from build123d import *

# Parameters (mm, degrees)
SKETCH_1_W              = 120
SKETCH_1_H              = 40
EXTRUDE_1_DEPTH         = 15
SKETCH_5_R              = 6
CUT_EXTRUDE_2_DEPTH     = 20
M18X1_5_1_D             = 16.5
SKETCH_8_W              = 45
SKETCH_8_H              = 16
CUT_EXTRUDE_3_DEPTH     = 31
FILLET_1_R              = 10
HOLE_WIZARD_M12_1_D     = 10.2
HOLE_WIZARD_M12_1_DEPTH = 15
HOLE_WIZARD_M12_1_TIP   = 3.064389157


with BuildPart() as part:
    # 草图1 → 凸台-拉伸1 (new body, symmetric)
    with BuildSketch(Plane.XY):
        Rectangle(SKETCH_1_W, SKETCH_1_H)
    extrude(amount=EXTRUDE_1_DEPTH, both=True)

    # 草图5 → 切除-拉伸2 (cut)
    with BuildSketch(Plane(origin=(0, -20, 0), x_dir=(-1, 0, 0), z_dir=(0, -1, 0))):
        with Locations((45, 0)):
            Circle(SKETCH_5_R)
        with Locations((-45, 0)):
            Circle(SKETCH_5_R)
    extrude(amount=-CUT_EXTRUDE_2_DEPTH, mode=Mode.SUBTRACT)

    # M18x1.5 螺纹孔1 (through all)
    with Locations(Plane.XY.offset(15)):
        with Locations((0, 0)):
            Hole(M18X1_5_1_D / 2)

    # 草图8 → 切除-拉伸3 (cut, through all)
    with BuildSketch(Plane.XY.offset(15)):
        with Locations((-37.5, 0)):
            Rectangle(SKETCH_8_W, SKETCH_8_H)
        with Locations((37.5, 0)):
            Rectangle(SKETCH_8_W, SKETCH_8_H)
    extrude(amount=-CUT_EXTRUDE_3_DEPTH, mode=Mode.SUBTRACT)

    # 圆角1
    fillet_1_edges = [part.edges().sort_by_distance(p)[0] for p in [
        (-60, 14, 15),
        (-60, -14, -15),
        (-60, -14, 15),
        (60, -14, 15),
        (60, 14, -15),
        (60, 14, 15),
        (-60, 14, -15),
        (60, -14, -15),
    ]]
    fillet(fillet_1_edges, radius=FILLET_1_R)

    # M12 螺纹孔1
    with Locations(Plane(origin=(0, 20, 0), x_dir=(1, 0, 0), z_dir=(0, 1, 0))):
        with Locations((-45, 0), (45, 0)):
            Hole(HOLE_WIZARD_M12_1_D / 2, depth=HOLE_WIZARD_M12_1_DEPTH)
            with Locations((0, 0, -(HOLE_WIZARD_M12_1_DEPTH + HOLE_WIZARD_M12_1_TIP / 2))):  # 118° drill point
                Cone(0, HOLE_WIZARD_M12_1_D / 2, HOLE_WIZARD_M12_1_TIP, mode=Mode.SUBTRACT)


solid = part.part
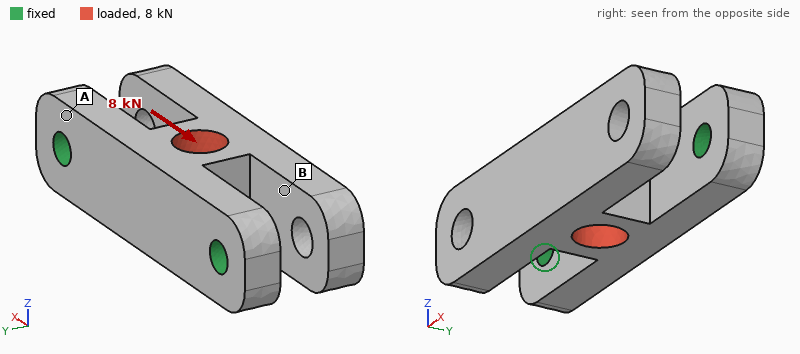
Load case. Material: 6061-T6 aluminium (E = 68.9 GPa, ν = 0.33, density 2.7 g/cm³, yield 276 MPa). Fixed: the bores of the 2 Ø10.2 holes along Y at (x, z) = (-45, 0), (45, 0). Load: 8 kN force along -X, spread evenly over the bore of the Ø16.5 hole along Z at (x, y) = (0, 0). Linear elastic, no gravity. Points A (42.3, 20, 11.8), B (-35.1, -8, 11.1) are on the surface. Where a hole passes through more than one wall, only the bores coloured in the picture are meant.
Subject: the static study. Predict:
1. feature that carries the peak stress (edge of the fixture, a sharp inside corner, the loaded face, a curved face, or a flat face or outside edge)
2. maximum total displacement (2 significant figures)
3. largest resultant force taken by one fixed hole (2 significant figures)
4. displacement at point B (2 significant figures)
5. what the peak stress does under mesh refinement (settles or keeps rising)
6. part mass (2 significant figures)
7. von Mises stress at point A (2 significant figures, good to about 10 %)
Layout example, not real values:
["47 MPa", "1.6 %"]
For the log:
["edge of the fixture", "73 µm", "4.4 kN", "48 µm", "keeps rising", "240 g", "16 MPa"]
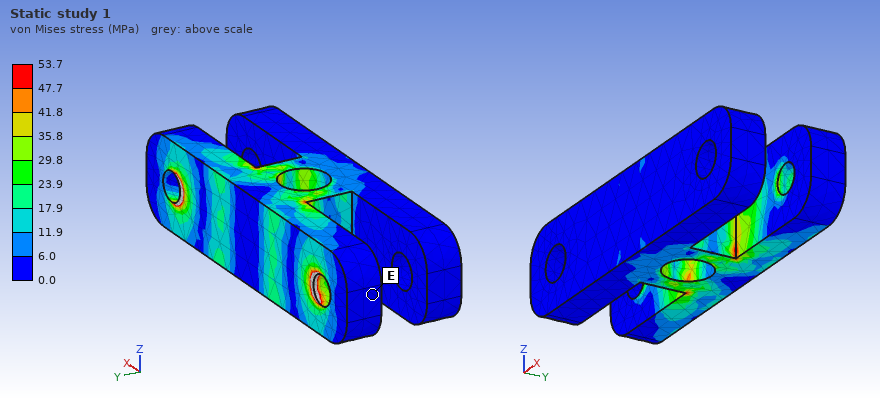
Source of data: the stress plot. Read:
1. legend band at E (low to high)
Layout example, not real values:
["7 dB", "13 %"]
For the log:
["0.0 to 6.0 MPa"]
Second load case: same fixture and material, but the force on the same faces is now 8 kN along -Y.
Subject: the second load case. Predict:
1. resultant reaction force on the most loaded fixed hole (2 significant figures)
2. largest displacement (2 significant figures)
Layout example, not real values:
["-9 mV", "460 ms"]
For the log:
["4.1 kN", "77 µm"]
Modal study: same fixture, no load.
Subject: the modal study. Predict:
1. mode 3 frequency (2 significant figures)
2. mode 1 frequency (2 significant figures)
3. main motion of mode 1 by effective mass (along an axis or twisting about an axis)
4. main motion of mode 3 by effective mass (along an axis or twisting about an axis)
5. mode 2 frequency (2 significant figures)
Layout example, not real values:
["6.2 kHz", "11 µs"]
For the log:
["3100 Hz", "2200 Hz", "along Z", "twisting about Y", "2700 Hz"]
